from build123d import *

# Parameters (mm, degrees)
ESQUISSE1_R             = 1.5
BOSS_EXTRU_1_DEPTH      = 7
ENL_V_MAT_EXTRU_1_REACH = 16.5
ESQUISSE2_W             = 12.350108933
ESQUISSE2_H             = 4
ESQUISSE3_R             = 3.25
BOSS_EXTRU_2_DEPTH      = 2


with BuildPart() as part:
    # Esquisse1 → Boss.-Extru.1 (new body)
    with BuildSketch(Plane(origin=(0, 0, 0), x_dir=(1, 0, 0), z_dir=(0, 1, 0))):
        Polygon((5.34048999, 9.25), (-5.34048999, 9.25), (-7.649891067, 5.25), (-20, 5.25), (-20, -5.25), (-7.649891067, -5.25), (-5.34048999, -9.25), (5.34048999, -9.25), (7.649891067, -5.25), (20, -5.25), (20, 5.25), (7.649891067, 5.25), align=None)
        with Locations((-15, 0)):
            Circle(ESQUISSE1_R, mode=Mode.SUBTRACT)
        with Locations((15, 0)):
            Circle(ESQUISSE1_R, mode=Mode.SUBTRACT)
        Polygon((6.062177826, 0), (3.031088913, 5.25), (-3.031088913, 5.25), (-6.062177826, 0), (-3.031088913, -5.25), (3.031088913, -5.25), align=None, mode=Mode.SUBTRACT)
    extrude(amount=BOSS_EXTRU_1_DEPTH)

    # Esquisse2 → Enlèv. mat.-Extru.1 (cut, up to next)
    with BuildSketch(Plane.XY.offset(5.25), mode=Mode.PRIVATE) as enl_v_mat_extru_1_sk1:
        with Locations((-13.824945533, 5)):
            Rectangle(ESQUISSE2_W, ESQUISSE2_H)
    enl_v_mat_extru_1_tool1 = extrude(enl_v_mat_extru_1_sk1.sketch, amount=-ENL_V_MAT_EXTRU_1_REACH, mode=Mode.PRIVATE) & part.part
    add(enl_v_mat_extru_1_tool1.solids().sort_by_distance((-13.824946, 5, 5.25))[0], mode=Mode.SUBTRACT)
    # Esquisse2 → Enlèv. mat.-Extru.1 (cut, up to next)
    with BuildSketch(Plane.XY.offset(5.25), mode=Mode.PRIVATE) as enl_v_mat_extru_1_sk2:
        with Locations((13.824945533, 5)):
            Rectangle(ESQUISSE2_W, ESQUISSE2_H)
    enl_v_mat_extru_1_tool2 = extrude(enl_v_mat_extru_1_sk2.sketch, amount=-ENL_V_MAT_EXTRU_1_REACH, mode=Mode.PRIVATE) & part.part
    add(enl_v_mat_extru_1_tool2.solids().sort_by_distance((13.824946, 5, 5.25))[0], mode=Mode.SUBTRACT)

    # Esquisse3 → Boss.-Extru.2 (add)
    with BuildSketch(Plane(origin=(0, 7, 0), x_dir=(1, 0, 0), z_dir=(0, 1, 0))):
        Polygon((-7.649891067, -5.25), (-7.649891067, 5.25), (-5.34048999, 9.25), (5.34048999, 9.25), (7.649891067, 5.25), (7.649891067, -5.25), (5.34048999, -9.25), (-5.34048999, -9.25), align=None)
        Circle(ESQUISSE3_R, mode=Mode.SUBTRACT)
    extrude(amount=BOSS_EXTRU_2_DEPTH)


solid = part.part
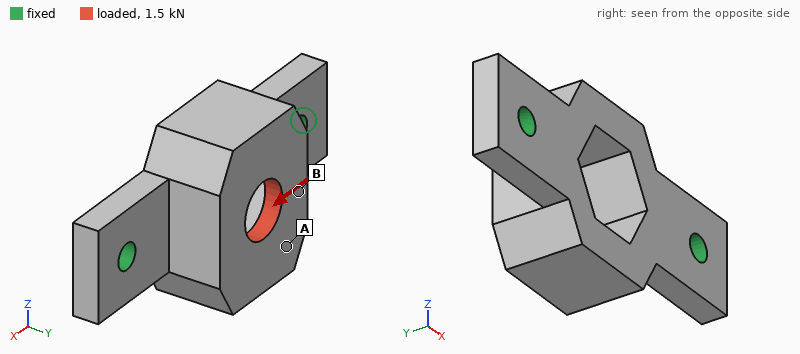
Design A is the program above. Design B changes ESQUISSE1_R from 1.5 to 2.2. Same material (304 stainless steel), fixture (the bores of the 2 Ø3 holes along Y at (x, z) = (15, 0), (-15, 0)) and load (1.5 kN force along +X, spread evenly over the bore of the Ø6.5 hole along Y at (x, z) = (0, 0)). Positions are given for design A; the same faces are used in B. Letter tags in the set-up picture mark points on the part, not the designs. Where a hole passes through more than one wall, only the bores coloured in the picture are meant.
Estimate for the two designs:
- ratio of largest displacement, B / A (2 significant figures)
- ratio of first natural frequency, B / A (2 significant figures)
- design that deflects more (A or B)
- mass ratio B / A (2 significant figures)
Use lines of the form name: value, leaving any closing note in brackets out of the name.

ratio of largest displacement, B / A: 0.87
ratio of first natural frequency, B / A: 1.1
design that deflects more: A
mass ratio B / A: 0.98
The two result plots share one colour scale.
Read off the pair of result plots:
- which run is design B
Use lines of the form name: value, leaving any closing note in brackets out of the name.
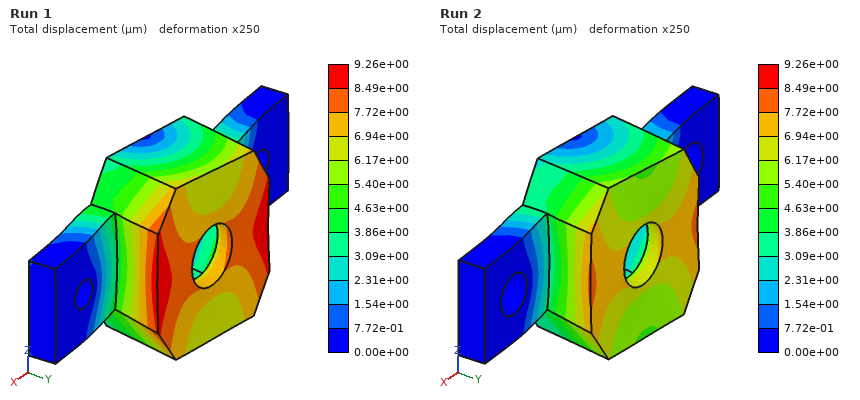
which run is design B: Run 2
